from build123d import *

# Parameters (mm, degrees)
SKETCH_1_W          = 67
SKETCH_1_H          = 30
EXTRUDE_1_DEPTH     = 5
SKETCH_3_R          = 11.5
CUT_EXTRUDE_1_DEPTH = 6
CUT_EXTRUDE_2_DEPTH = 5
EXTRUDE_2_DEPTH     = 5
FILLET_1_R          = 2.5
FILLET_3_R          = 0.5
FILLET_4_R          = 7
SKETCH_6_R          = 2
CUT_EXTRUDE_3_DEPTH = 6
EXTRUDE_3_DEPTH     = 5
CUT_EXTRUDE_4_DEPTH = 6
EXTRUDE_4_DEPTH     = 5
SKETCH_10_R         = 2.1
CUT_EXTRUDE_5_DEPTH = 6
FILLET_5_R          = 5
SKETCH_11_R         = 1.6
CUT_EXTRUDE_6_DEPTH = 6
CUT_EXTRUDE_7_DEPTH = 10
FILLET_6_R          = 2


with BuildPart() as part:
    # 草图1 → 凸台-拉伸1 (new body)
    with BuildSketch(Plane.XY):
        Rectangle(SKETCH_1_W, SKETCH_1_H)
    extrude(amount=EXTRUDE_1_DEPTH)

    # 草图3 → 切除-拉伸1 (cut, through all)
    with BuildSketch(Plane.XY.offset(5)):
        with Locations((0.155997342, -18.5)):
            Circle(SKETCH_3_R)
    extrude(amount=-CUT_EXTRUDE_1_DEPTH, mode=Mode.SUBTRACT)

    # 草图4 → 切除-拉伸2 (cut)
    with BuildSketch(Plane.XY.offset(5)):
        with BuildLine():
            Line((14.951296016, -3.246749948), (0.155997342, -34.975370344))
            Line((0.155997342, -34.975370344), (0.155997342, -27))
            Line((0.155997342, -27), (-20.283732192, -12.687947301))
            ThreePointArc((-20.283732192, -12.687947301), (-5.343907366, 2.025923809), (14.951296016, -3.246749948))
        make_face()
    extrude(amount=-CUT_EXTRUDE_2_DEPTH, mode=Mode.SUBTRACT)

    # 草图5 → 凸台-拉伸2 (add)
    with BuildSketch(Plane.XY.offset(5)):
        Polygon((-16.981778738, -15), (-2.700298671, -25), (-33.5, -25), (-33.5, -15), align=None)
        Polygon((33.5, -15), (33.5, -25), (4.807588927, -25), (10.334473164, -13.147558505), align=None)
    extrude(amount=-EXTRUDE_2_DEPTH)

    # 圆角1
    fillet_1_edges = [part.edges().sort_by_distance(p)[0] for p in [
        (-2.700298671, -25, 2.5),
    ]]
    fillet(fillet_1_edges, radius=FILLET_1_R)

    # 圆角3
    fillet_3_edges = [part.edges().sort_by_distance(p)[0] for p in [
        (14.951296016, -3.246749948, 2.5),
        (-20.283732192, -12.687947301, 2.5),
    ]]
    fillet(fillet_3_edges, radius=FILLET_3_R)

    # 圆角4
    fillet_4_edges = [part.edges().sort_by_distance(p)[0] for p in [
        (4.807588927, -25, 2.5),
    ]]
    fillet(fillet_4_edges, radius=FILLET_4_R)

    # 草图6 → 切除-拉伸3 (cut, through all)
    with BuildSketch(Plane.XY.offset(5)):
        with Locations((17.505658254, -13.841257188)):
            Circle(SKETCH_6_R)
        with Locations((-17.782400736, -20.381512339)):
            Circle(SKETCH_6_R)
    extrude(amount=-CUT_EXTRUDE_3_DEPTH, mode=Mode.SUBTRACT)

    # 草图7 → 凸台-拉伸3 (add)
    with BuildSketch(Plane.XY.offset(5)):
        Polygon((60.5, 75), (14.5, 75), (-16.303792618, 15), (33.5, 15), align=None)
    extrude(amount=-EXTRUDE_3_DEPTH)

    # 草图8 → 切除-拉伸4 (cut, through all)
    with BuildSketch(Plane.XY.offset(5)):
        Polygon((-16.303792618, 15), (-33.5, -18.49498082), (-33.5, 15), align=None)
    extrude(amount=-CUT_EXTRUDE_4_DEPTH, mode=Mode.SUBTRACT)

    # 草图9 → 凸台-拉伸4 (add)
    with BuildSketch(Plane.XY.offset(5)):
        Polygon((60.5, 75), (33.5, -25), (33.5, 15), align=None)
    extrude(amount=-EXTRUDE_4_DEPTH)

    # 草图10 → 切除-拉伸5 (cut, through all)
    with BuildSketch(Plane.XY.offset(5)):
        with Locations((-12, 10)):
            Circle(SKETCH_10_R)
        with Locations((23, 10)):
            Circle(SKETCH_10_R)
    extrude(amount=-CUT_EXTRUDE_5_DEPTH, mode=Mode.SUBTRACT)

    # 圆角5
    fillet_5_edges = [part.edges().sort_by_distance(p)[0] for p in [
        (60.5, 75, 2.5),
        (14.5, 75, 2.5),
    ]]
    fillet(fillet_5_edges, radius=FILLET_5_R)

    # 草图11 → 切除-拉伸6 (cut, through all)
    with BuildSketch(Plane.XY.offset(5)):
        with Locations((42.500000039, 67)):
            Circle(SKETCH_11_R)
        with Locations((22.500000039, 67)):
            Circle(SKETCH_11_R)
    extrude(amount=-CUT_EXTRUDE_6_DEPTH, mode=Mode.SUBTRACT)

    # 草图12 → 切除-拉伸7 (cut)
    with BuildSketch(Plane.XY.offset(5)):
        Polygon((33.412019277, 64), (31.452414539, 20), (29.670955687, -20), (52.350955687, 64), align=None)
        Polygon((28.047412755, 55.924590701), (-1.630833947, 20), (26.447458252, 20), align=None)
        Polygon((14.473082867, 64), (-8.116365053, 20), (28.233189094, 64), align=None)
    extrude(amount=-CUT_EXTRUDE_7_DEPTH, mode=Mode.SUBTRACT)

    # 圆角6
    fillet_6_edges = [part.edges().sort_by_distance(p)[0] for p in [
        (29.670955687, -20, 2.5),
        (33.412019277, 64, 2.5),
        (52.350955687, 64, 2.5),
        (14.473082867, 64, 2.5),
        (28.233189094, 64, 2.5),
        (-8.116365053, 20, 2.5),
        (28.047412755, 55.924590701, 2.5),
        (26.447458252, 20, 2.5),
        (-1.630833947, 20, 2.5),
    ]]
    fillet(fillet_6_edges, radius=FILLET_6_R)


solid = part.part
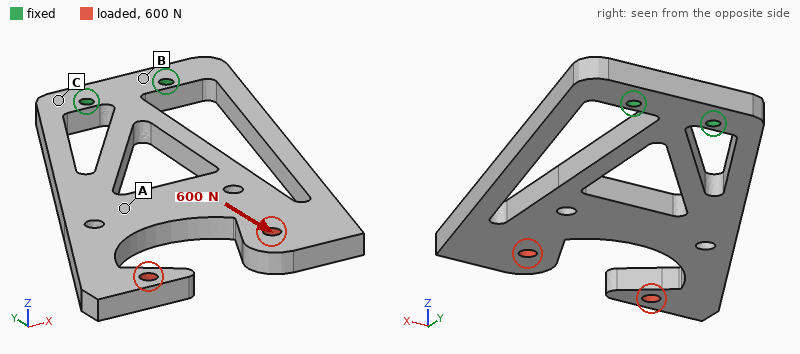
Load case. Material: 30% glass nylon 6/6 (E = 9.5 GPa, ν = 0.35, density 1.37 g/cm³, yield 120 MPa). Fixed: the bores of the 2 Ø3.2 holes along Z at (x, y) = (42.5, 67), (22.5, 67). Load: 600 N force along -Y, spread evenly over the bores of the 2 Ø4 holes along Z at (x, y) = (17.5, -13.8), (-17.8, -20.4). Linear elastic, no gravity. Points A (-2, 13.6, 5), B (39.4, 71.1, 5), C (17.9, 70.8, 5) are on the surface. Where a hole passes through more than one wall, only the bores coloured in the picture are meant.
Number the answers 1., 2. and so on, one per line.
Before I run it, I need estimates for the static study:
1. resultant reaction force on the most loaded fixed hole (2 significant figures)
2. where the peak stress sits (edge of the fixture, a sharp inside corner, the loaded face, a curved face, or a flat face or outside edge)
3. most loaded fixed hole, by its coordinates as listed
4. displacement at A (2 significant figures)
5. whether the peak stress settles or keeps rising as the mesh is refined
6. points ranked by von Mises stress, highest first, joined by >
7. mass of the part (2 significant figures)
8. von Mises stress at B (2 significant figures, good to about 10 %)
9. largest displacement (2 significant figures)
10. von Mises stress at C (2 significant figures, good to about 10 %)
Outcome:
1. 1.1 kN
2. edge of the fixture
3. (22.5, 67)
4. 0.80 mm
5. keeps rising
6. C > B > A
7. 24 g
8. 15 MPa
9. 1.3 mm
10. 27 MPa
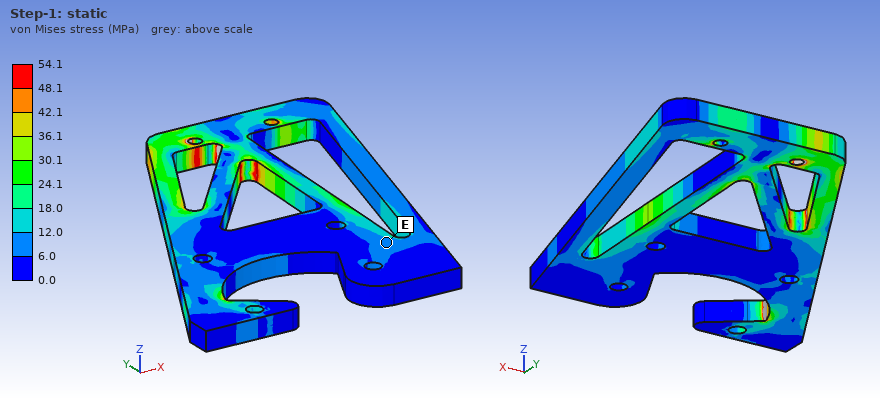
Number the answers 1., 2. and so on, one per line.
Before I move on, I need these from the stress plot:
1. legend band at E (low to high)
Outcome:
1. 6.0 to 12.0 MPa
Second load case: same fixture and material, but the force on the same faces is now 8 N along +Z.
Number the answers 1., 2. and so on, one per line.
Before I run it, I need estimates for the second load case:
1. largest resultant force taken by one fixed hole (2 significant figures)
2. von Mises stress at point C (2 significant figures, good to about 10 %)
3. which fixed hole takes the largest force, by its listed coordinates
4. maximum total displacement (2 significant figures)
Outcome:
1. 17 N
2. 3.1 MPa
3. (22.5, 67)
4. 1.4 mm
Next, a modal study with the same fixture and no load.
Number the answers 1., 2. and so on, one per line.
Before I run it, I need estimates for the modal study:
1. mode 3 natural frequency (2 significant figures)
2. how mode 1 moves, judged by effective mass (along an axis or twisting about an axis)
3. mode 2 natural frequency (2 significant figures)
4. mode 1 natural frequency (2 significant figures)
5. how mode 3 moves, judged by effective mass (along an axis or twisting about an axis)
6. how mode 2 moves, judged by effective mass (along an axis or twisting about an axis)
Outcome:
1. 640 Hz
2. along Z
3. 390 Hz
4. 150 Hz
5. along X
6. twisting about Y
